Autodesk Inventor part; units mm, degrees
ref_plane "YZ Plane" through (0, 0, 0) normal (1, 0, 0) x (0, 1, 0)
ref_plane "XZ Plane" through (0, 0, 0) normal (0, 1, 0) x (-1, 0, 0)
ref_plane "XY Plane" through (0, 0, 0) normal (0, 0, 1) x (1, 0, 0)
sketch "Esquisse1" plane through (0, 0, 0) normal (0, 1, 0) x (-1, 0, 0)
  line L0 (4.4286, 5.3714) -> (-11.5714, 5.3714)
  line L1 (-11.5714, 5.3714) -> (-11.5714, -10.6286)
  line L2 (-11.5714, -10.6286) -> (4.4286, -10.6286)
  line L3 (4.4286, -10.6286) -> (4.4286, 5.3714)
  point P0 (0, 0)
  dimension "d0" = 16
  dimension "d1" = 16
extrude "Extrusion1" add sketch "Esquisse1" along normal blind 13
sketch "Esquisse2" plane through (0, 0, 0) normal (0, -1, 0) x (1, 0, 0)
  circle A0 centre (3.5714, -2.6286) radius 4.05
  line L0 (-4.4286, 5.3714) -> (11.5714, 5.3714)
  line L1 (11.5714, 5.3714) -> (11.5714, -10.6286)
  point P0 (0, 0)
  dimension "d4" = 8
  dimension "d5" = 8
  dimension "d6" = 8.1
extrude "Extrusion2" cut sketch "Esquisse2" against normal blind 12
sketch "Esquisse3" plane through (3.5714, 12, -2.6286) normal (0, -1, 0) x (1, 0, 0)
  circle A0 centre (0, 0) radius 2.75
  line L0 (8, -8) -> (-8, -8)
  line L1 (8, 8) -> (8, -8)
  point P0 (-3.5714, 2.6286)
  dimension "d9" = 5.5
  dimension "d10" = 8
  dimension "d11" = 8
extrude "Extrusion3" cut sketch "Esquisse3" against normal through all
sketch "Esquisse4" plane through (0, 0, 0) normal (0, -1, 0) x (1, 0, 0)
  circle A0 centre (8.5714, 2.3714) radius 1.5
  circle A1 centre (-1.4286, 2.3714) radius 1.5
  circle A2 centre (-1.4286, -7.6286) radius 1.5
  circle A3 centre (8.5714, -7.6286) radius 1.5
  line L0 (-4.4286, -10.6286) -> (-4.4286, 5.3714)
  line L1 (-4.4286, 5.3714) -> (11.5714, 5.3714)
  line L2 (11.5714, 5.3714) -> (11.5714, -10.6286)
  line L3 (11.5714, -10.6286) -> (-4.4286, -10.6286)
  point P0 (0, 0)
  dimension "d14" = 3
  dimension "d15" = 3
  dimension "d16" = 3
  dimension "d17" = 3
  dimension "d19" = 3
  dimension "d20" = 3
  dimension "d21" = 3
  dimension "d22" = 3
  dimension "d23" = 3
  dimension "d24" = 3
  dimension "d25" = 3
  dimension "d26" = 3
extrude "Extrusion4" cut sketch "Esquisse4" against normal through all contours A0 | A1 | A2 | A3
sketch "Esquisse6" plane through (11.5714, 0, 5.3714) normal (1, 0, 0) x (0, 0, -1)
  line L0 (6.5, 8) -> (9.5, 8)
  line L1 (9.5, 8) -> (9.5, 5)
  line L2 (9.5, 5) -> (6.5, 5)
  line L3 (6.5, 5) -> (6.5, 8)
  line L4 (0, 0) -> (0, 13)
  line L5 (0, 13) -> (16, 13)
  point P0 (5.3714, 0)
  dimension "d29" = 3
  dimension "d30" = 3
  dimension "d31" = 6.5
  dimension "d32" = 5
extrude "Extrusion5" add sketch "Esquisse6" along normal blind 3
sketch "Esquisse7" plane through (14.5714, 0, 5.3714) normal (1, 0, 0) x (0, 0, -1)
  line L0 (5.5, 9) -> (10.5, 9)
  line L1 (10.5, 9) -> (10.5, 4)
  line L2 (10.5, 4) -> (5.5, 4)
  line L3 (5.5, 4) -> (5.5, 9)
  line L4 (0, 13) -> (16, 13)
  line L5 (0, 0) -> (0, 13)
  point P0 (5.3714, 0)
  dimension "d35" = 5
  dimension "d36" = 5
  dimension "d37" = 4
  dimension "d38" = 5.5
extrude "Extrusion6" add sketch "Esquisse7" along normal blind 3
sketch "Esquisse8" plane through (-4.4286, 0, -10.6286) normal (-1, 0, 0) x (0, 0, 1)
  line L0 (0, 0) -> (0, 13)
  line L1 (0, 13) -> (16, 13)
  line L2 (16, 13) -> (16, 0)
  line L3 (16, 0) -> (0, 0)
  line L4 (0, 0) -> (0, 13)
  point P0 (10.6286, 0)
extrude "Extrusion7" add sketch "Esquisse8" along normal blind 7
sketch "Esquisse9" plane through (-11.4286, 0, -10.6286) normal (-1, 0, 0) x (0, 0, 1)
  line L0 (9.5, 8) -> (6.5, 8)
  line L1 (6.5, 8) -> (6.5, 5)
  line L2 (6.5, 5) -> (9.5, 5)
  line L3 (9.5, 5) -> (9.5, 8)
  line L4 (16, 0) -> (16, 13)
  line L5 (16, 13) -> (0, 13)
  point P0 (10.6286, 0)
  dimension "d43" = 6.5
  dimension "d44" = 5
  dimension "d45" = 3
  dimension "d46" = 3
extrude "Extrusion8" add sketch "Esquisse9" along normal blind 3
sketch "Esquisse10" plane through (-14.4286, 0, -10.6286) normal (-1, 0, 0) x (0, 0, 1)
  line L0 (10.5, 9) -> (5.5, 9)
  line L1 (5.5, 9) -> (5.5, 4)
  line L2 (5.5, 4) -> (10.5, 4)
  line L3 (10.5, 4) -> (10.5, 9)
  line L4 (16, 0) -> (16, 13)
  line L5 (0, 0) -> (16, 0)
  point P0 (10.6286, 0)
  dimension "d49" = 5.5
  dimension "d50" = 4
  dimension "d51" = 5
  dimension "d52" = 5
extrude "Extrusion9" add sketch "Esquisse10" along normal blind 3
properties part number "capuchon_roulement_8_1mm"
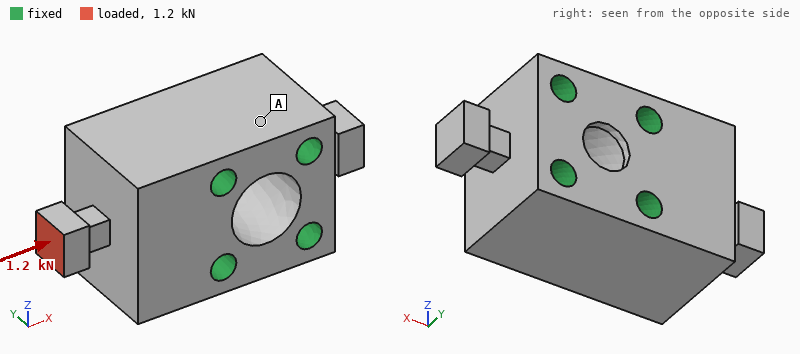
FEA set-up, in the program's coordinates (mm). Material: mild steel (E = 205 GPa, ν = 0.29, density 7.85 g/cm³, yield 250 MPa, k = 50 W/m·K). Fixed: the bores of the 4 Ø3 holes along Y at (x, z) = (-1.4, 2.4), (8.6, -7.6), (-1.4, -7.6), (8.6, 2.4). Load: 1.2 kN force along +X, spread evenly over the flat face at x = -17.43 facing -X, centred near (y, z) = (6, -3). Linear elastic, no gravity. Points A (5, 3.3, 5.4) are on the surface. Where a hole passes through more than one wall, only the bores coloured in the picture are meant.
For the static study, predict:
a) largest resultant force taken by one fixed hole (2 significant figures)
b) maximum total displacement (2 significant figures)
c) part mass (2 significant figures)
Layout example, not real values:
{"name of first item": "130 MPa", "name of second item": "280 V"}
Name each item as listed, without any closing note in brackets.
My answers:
{"largest resultant force taken by one fixed hole": "630 N", "maximum total displacement": "4.4 µm", "part mass": "31 g"}
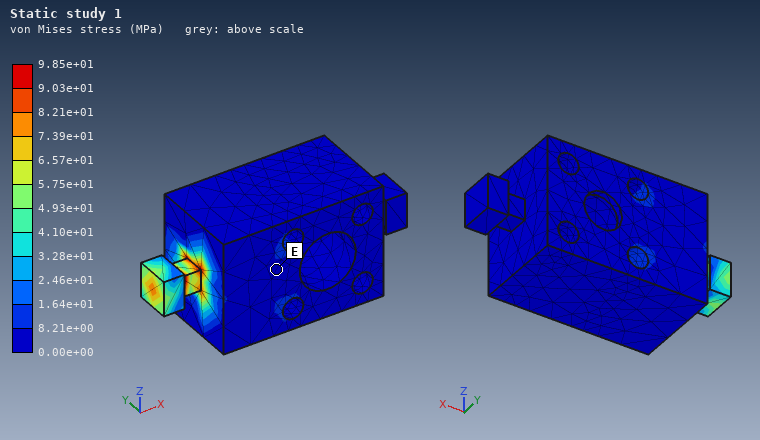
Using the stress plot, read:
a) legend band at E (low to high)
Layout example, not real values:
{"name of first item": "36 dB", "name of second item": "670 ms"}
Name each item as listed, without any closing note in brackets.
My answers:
{"legend band at E": "0.00e+00 to 8.21e+00 MPa"}
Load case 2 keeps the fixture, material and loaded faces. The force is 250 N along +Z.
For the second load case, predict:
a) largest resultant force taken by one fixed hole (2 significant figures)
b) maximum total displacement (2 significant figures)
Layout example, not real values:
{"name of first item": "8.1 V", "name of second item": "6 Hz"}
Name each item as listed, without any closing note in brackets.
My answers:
{"largest resultant force taken by one fixed hole": "350 N", "maximum total displacement": "21 µm"}
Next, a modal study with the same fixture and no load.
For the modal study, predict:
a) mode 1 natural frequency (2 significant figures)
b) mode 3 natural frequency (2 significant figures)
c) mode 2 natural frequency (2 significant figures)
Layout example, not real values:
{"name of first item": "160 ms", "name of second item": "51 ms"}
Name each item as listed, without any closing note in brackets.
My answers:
{"mode 1 natural frequency": "30 kHz", "mode 3 natural frequency": "30 kHz", "mode 2 natural frequency": "30 kHz"}
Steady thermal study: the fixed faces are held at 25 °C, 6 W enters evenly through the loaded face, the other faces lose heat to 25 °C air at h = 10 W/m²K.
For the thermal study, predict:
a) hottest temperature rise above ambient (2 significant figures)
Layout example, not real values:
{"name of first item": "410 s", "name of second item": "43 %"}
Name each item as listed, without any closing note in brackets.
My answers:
{"hottest temperature rise above ambient": "76 K"}
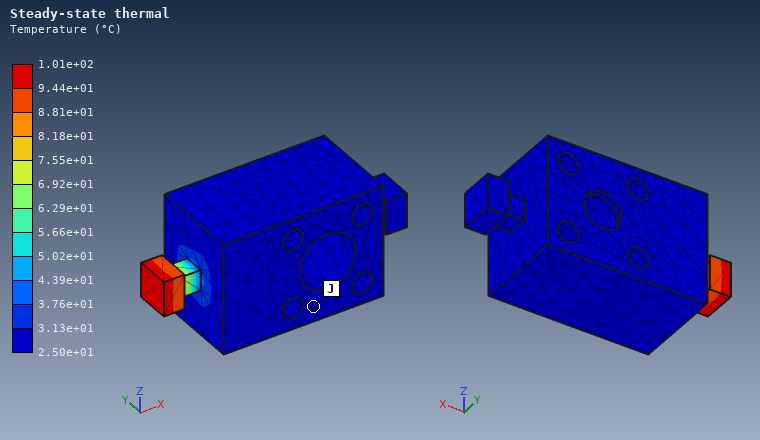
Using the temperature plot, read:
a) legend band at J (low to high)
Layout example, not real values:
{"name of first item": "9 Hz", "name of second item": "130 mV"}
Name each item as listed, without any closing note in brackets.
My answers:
{"legend band at J": "2.50e+01 to 3.13e+01 °C"}
